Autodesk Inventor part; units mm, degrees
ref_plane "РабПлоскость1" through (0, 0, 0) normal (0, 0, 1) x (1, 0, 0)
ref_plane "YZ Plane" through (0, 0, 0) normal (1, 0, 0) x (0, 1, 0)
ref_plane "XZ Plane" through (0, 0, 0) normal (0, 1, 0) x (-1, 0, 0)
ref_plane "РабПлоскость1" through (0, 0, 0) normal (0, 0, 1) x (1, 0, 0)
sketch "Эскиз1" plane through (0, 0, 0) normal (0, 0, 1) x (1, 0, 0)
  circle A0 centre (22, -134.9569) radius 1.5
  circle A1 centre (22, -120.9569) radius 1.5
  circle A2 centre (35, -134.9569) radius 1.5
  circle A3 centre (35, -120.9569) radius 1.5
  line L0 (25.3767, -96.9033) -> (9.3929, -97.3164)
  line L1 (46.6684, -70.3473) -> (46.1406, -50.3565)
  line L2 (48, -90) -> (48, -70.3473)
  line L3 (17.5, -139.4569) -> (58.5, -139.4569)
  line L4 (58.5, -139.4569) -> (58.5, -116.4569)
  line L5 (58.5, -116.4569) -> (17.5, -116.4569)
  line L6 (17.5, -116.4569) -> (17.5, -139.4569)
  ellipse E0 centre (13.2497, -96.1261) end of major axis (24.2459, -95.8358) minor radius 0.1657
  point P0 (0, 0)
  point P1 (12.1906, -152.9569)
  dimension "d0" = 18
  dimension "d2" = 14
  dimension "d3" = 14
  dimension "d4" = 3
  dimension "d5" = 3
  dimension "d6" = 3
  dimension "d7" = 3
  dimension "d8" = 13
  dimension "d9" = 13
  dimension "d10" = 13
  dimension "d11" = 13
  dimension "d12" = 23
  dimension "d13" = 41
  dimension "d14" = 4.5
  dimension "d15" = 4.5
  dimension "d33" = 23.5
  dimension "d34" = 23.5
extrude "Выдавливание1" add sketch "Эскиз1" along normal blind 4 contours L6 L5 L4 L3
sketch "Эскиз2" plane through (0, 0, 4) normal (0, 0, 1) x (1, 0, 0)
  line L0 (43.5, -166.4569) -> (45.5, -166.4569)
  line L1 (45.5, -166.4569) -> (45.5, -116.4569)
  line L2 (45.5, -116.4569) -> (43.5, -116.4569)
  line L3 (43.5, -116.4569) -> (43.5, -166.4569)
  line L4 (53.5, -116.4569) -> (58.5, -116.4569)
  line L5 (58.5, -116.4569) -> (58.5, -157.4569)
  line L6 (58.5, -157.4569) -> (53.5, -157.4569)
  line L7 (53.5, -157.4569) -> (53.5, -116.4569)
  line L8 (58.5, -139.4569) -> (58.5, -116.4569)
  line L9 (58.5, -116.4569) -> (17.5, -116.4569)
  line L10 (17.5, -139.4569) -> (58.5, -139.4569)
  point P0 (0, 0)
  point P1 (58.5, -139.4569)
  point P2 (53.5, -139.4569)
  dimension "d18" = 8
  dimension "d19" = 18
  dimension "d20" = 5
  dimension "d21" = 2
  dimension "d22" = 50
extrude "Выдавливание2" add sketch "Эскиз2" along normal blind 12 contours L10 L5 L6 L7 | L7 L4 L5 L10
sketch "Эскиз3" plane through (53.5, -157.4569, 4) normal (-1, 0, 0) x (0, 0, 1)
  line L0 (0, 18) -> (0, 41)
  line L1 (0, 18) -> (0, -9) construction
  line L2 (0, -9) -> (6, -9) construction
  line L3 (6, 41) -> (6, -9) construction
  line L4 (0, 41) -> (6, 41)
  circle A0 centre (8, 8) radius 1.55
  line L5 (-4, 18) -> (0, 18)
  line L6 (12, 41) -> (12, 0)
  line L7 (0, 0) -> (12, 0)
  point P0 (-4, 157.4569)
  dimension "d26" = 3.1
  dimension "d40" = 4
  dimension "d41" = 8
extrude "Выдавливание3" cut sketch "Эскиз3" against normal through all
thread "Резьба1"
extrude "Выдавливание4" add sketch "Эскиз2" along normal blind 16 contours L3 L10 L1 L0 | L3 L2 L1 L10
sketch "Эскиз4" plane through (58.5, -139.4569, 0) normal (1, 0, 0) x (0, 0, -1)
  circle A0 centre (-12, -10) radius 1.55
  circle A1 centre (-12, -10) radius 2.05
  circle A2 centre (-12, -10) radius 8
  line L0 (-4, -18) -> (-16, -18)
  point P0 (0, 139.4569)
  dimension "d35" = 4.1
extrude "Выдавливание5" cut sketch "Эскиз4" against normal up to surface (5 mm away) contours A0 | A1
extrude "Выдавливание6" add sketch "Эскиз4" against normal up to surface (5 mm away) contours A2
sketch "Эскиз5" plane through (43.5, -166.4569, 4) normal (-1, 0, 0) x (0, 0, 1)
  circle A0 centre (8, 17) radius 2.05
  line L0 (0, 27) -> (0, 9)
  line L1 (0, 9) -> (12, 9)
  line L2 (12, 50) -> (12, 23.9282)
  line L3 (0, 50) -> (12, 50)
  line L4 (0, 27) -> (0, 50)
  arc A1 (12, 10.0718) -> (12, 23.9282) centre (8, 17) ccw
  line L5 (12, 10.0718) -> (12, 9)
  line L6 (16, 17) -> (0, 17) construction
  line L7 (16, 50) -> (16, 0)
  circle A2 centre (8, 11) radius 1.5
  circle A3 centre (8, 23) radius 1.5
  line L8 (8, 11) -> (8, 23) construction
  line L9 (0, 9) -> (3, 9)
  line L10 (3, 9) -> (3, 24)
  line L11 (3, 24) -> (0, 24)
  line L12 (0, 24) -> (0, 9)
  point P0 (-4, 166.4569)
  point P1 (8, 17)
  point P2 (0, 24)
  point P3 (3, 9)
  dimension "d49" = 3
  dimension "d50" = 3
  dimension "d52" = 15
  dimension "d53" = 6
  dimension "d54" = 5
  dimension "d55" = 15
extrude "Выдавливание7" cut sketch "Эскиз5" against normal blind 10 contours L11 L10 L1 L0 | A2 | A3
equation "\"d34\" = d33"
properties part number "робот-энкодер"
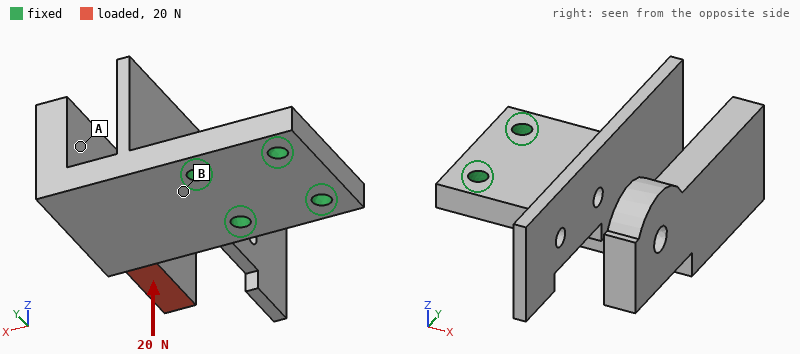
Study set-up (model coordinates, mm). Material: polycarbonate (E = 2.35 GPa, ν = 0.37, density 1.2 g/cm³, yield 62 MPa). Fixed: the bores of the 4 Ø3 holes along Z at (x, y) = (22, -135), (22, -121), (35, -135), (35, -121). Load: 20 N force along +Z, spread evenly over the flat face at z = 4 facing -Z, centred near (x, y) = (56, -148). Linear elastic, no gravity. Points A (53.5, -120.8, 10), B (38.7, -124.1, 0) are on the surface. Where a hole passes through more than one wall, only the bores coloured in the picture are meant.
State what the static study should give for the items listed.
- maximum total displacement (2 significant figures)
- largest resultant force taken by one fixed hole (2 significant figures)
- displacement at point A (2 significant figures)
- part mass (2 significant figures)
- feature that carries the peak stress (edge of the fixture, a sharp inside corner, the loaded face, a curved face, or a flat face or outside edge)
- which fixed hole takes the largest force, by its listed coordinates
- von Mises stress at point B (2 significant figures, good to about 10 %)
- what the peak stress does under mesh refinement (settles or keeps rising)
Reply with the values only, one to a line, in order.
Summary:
0.68 mm
39 N
0.16 mm
9.3 g
edge of the fixture
(35, -135)
4.3 MPa
keeps rising
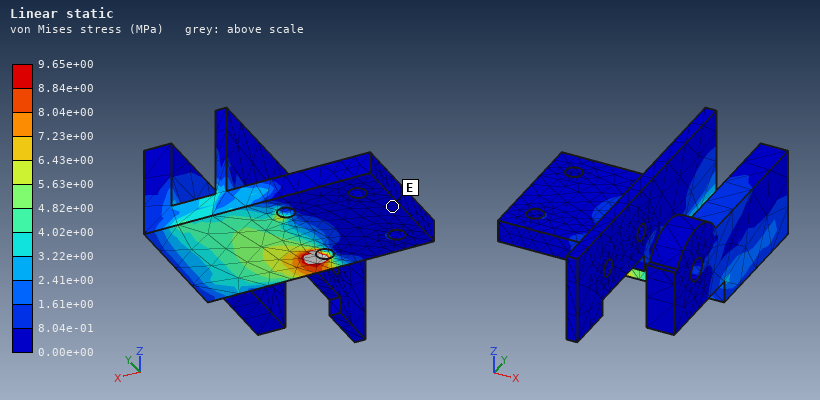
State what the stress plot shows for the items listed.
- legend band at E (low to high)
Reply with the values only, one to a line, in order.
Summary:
0.00e+00 to 8.04e-01 MPa
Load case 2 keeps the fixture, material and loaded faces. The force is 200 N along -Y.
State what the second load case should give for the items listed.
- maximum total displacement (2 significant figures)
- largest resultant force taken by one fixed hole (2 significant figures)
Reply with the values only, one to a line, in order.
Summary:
0.35 mm
260 N
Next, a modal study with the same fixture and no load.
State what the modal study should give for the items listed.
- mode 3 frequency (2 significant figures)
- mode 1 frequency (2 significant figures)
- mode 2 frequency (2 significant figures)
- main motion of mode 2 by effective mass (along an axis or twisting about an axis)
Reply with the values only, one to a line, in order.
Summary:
970 Hz
390 Hz
610 Hz
along Z
